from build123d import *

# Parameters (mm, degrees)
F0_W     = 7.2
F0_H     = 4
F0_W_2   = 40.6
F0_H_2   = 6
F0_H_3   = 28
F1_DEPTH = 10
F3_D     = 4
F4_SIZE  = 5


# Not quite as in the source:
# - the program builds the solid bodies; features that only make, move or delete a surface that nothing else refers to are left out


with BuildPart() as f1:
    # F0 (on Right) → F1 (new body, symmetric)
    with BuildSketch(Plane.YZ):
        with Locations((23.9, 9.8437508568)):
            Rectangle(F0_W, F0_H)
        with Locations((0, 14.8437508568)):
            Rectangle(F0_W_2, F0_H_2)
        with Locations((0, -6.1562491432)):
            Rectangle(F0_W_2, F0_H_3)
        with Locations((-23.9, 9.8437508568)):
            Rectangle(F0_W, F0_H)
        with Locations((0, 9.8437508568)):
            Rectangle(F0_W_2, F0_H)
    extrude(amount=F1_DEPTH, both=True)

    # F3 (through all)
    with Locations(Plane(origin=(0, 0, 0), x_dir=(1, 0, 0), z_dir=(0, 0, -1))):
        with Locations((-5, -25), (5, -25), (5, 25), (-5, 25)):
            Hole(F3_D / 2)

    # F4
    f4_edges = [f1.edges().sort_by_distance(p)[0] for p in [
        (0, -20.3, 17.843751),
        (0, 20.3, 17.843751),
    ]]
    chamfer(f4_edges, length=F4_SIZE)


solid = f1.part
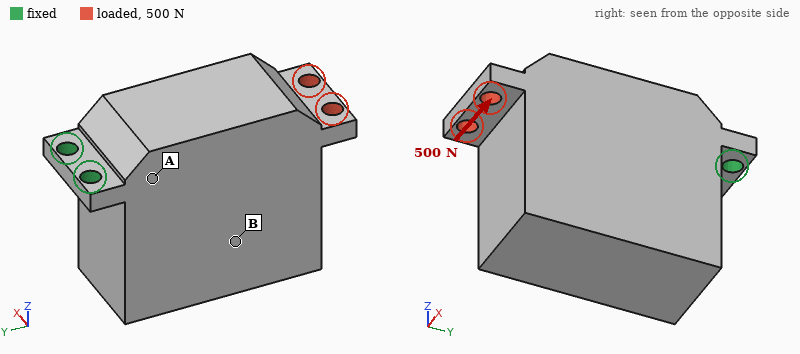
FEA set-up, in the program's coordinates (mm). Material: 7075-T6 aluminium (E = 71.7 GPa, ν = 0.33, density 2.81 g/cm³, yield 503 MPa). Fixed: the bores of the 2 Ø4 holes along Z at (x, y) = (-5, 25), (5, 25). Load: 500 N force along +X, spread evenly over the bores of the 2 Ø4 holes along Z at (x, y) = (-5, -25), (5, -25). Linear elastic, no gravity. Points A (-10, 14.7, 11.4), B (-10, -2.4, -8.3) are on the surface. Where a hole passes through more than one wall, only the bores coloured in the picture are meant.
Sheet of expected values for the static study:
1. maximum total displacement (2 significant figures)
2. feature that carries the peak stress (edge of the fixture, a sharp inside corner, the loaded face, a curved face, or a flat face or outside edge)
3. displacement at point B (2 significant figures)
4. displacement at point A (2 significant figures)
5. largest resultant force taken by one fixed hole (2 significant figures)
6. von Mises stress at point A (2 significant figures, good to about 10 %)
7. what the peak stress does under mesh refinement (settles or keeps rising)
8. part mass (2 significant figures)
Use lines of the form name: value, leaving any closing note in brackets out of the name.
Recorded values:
maximum total displacement: 73 µm
feature that carries the peak stress: edge of the fixture
displacement at point B: 33 µm
displacement at point A: 14 µm
largest resultant force taken by one fixed hole: 2.0 kN
von Mises stress at point A: 29 MPa
what the peak stress does under mesh refinement: keeps rising
part mass: 88 g
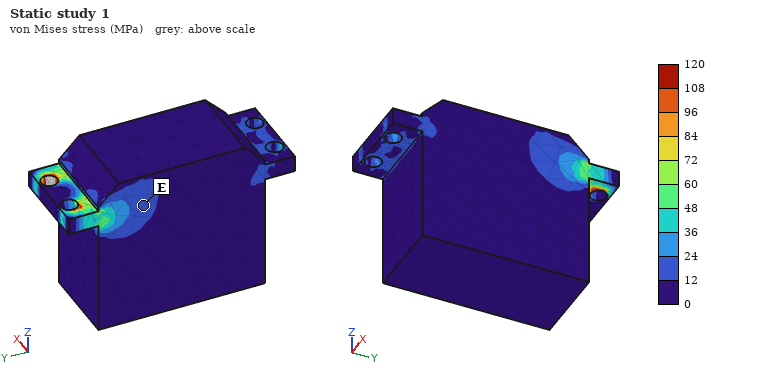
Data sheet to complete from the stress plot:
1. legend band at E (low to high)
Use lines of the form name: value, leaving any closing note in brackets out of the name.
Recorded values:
legend band at E: 12 to 24 MPa
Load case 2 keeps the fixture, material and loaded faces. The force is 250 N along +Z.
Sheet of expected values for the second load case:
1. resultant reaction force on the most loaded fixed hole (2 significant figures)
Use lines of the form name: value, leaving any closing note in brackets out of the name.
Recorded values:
resultant reaction force on the most loaded fixed hole: 130 N
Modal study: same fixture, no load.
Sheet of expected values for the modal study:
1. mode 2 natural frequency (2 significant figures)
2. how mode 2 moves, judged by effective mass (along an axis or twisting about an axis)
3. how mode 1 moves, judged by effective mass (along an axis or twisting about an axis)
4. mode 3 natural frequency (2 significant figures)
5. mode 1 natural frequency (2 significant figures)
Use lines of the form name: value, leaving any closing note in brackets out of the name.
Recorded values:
mode 2 natural frequency: 2300 Hz
how mode 2 moves, judged by effective mass: along X
how mode 1 moves, judged by effective mass: along Z
mode 3 natural frequency: 4300 Hz
mode 1 natural frequency: 720 Hz
